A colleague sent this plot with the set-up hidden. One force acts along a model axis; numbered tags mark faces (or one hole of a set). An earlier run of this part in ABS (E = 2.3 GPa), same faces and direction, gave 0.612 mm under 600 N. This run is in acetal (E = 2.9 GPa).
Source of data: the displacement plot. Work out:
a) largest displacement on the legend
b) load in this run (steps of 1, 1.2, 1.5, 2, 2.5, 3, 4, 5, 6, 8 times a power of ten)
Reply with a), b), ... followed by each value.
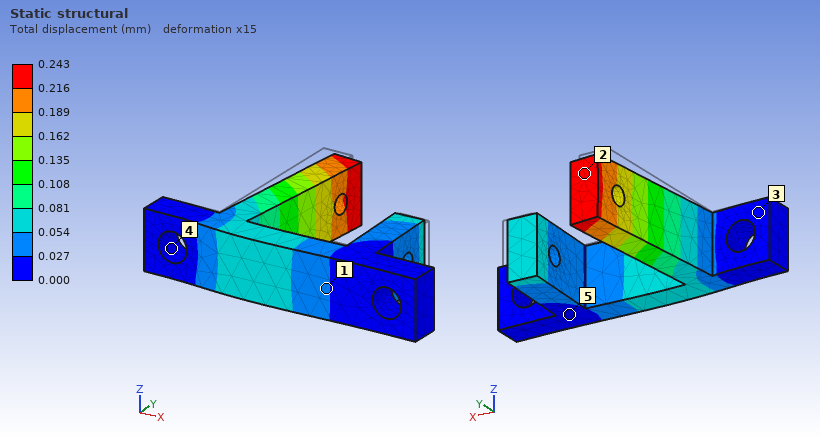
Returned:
a) 0.243 mm
b) 300 N
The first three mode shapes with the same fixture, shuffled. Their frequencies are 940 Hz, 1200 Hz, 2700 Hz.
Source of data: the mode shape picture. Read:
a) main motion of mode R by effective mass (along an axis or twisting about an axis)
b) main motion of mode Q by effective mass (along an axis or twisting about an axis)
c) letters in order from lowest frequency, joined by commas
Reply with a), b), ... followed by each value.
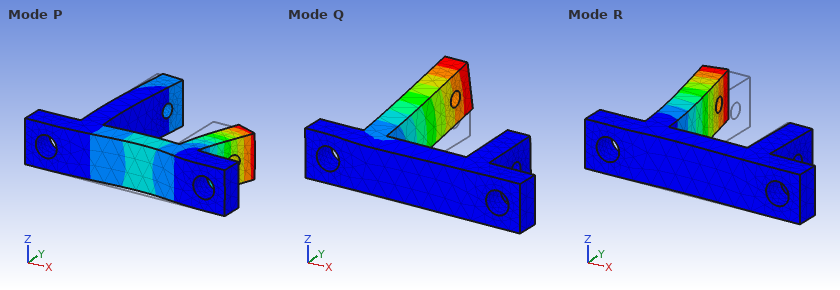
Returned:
a) along X
b) along Z
c) R, Q, P
